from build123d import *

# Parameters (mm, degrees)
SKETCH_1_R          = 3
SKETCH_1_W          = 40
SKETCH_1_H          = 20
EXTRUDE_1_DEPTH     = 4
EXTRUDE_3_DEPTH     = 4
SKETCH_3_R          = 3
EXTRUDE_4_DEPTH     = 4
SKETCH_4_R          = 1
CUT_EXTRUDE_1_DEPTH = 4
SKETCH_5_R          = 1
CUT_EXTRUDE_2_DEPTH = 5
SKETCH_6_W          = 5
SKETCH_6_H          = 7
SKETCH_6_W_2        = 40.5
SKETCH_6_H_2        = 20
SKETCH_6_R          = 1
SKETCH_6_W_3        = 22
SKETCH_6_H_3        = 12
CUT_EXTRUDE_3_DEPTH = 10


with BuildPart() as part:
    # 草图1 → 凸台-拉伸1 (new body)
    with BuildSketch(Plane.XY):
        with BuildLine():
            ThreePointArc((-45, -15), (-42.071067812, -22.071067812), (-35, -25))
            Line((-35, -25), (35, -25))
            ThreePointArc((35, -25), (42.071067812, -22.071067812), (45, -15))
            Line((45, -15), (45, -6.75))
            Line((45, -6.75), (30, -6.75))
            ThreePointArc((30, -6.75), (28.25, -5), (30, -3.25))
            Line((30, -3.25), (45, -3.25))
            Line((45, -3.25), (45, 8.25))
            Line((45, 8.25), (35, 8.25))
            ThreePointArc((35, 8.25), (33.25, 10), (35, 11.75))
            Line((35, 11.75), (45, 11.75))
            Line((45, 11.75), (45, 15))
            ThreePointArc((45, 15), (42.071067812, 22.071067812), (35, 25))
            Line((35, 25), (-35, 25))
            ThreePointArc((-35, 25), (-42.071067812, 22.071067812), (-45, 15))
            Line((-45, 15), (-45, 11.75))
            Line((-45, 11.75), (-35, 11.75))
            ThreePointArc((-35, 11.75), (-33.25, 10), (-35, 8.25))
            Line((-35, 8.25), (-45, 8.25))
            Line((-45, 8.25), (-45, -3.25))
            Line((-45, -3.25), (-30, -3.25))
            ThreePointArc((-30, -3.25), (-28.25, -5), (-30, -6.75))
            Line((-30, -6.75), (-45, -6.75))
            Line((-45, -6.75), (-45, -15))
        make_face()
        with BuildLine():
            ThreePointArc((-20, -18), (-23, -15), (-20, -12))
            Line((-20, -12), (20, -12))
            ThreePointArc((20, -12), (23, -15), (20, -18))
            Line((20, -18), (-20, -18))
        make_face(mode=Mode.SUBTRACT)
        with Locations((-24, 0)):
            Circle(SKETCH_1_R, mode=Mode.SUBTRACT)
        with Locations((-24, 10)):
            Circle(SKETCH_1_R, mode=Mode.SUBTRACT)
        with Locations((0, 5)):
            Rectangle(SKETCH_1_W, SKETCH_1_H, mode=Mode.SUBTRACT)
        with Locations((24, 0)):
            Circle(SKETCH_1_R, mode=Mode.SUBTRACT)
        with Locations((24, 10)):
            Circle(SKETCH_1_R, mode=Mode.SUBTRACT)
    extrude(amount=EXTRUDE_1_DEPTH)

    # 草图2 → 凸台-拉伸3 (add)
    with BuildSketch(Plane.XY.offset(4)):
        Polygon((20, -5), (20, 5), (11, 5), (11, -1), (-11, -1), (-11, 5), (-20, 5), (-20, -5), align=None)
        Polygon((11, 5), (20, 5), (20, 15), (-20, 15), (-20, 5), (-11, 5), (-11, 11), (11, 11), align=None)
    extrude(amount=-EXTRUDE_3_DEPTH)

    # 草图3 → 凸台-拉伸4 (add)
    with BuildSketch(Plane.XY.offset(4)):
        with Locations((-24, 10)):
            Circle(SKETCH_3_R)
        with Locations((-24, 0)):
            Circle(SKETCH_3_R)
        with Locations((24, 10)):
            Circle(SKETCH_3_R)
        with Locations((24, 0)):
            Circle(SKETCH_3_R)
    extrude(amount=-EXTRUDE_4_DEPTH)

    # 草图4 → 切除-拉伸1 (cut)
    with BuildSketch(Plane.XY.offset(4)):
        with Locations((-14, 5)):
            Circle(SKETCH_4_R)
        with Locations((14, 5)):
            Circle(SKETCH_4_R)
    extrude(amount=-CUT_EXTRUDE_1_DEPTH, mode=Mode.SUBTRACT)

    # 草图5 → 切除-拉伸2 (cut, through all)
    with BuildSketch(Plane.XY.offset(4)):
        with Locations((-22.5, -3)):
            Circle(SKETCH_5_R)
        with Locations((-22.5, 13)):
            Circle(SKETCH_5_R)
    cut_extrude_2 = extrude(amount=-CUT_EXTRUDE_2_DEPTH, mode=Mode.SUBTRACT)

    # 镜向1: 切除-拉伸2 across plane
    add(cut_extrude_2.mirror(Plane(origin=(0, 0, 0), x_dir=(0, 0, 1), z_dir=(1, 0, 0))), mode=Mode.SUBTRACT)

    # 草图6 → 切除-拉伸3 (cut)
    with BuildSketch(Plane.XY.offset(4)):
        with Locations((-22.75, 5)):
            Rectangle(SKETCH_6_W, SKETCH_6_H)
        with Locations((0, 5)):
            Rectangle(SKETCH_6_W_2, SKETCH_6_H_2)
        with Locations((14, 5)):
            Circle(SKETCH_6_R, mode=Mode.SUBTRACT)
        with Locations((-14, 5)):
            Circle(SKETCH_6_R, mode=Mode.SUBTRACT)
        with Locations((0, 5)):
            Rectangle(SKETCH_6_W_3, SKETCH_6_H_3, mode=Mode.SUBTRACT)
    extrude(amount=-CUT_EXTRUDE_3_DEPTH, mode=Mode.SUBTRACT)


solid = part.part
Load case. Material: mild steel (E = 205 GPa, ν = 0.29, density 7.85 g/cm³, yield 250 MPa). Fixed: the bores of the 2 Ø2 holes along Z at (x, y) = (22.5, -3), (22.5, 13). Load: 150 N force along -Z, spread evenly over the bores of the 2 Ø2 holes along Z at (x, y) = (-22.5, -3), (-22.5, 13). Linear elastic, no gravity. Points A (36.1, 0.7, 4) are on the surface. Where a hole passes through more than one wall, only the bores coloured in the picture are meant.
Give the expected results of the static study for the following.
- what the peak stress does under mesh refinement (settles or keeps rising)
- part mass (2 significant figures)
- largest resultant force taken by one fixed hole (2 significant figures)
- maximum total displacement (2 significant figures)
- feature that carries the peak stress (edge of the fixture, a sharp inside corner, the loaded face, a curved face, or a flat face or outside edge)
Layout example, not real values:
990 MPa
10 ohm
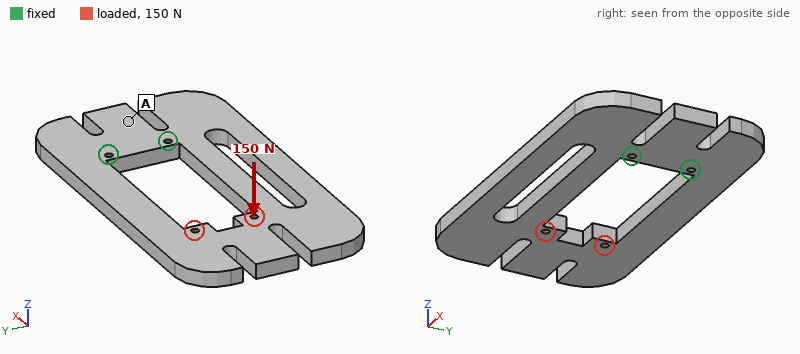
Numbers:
keeps rising
97 g
79 N
0.44 mm
edge of the fixture
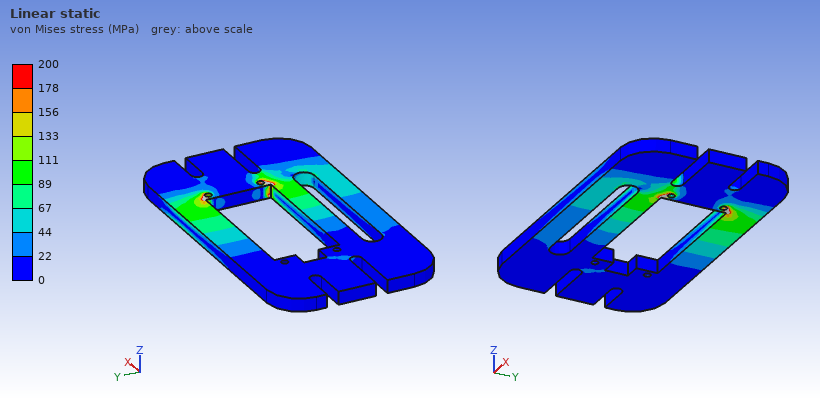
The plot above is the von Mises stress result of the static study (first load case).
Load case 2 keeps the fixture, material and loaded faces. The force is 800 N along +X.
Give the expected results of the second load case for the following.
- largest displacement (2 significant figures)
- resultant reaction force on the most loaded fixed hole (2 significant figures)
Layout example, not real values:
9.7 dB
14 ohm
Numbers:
9.6 µm
460 N
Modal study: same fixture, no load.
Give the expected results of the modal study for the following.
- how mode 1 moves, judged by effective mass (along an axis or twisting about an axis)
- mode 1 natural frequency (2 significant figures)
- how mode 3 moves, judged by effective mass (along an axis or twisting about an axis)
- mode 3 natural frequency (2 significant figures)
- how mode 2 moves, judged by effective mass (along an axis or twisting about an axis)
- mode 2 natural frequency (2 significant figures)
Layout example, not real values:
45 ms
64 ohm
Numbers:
along Z
480 Hz
along Y
1600 Hz
twisting about X
1300 Hz
